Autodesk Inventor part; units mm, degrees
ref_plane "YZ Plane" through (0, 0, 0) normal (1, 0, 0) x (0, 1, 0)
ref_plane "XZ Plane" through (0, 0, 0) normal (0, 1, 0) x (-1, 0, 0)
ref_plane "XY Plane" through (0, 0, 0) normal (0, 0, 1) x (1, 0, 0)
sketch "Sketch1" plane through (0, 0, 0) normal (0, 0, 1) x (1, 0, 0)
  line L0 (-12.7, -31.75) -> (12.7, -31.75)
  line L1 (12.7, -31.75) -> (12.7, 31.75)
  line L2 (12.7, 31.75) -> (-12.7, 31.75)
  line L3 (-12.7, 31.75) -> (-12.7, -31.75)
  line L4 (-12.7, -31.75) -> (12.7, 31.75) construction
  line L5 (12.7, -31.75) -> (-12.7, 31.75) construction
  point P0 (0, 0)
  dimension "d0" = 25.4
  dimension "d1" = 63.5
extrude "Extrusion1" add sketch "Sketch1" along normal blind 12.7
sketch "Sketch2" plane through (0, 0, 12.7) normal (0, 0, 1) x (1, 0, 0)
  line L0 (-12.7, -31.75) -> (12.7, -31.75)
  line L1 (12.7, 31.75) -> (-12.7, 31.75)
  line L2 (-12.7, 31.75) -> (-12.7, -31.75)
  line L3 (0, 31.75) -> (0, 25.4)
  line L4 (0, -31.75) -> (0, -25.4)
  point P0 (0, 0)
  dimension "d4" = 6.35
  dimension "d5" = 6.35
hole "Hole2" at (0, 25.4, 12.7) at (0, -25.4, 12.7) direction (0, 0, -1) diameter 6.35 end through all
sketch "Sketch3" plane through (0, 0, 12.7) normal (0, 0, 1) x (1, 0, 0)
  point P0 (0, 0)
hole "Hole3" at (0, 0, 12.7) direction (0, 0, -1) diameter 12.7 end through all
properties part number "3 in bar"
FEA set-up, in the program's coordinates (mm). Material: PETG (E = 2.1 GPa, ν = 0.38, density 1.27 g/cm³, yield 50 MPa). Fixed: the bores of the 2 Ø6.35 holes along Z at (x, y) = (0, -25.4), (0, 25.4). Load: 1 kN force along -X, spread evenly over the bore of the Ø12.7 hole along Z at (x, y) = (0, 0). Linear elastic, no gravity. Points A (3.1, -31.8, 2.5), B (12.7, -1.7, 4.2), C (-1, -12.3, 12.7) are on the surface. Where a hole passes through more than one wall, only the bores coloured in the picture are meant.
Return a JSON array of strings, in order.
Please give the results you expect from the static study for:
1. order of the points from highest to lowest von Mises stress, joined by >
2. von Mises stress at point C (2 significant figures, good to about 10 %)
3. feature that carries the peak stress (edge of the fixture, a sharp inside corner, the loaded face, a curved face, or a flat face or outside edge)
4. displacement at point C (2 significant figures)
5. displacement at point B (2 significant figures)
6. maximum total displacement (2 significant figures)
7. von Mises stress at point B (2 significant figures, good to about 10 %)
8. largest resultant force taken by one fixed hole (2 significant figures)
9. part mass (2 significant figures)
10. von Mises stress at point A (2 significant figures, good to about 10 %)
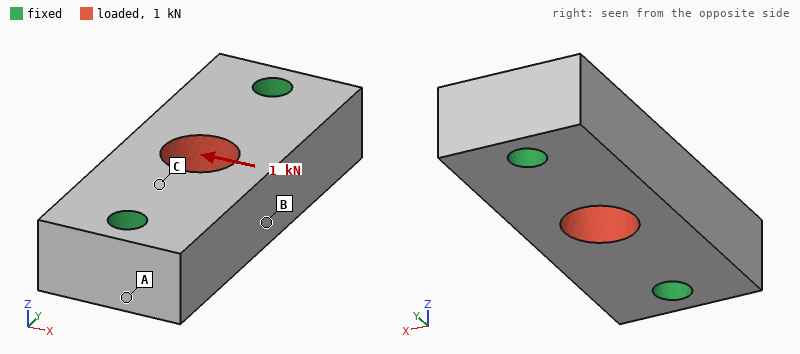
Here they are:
["B > C > A", "3.9 MPa", "edge of the fixture", "56 µm", "86 µm", "98 µm", "7.4 MPa", "500 N", "23 g", "1.8 MPa"]
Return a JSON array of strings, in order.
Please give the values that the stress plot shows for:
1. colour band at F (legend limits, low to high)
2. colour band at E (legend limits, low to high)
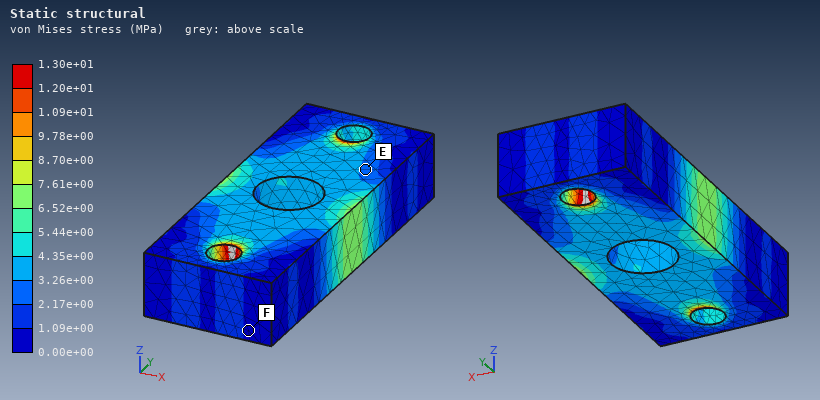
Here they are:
["0.00e+00 to 1.09e+00 MPa", "2.17e+00 to 3.26e+00 MPa"]
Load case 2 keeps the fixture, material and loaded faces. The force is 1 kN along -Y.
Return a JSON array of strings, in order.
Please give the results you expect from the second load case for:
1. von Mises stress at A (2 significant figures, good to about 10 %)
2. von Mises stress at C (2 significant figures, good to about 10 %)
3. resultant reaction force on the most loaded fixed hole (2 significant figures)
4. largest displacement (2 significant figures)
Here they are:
["1.4 MPa", "2.5 MPa", "500 N", "25 µm"]
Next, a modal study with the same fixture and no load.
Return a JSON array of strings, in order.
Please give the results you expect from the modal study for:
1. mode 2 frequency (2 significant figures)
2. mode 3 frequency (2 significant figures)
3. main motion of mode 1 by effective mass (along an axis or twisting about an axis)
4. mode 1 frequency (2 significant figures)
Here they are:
["5600 Hz", "5800 Hz", "along Z", "4800 Hz"]
